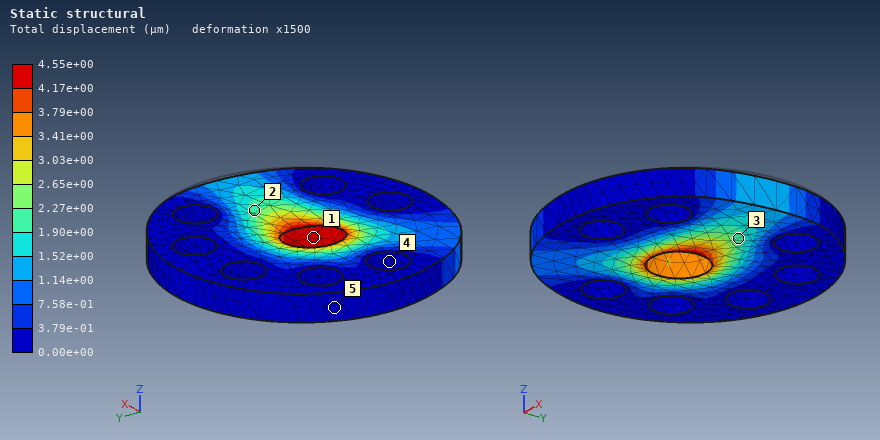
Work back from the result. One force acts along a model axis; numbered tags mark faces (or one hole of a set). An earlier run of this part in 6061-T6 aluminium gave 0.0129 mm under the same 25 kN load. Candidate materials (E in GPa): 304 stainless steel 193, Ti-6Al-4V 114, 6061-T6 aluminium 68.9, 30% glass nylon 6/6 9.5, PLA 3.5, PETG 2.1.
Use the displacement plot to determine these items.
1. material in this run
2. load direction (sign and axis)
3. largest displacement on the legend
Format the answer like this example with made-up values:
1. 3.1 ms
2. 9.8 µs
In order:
1. 304 stainless steel
2. -X
3. 4.55e+00 µm
